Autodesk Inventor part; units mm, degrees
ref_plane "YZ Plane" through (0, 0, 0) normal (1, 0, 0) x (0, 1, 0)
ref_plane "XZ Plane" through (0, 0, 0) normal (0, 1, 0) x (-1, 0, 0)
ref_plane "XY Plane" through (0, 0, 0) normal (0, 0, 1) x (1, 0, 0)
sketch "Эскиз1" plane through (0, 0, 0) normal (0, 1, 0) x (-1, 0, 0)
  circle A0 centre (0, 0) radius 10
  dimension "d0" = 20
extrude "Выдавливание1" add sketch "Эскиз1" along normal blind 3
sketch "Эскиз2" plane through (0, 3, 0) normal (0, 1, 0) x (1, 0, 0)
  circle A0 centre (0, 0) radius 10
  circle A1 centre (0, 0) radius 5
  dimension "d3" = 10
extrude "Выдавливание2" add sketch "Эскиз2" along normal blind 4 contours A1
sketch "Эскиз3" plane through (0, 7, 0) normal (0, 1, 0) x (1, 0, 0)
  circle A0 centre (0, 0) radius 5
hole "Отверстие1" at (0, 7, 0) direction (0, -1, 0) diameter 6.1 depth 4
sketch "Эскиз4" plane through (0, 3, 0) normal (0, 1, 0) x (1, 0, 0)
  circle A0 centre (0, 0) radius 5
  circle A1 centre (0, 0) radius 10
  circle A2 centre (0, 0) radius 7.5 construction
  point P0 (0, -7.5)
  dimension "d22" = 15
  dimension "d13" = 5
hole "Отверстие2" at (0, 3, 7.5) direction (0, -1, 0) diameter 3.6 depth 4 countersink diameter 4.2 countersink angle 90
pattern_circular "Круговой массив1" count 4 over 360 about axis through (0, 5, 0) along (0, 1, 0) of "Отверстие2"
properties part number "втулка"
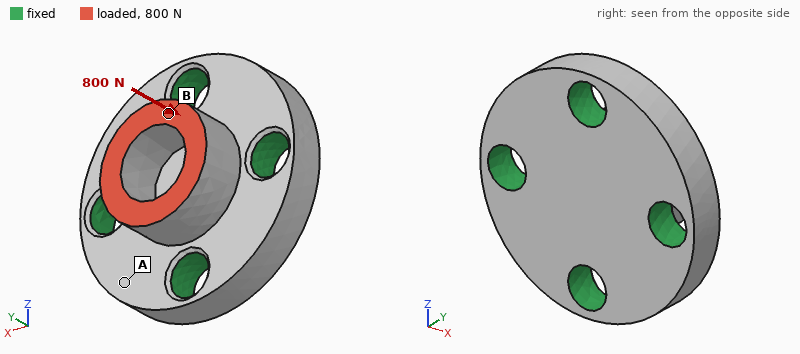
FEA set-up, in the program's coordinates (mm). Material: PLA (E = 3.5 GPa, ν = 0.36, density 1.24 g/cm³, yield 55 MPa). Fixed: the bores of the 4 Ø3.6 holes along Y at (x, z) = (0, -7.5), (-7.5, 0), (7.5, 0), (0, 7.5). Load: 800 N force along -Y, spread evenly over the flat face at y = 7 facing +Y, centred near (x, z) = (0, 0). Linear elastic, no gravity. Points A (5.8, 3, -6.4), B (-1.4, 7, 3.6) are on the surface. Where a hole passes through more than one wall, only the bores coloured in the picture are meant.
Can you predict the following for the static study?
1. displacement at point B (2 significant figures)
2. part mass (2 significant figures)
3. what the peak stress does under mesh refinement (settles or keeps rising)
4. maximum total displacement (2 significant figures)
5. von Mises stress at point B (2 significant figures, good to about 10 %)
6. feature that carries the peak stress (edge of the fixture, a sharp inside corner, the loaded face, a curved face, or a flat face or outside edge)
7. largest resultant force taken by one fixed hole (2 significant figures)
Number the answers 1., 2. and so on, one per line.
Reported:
1. 40 µm
2. 1.3 g
3. keeps rising
4. 44 µm
5. 16 MPa
6. edge of the fixture
7. 210 N
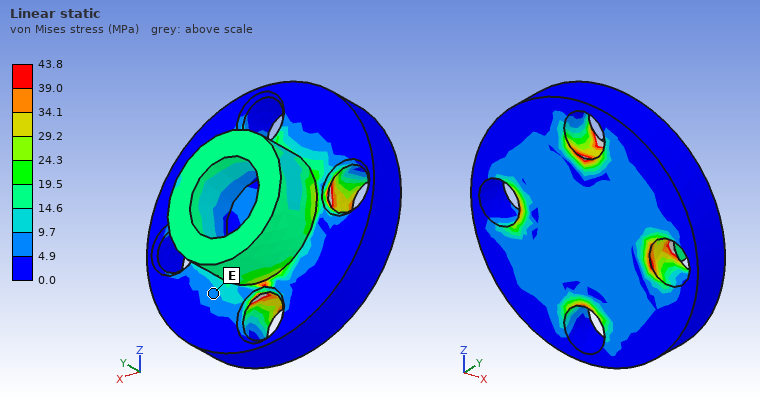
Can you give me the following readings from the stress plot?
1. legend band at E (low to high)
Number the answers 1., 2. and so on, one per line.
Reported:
1. 4.9 to 9.7 MPa
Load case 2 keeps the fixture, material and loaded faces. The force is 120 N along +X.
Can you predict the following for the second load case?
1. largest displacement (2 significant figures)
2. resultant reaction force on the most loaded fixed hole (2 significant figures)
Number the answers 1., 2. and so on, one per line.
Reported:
1. 30 µm
2. 62 N
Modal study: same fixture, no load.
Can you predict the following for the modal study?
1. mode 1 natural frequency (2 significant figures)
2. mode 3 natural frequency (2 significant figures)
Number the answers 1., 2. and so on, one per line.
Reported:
1. 32 kHz
2. 34 kHz
